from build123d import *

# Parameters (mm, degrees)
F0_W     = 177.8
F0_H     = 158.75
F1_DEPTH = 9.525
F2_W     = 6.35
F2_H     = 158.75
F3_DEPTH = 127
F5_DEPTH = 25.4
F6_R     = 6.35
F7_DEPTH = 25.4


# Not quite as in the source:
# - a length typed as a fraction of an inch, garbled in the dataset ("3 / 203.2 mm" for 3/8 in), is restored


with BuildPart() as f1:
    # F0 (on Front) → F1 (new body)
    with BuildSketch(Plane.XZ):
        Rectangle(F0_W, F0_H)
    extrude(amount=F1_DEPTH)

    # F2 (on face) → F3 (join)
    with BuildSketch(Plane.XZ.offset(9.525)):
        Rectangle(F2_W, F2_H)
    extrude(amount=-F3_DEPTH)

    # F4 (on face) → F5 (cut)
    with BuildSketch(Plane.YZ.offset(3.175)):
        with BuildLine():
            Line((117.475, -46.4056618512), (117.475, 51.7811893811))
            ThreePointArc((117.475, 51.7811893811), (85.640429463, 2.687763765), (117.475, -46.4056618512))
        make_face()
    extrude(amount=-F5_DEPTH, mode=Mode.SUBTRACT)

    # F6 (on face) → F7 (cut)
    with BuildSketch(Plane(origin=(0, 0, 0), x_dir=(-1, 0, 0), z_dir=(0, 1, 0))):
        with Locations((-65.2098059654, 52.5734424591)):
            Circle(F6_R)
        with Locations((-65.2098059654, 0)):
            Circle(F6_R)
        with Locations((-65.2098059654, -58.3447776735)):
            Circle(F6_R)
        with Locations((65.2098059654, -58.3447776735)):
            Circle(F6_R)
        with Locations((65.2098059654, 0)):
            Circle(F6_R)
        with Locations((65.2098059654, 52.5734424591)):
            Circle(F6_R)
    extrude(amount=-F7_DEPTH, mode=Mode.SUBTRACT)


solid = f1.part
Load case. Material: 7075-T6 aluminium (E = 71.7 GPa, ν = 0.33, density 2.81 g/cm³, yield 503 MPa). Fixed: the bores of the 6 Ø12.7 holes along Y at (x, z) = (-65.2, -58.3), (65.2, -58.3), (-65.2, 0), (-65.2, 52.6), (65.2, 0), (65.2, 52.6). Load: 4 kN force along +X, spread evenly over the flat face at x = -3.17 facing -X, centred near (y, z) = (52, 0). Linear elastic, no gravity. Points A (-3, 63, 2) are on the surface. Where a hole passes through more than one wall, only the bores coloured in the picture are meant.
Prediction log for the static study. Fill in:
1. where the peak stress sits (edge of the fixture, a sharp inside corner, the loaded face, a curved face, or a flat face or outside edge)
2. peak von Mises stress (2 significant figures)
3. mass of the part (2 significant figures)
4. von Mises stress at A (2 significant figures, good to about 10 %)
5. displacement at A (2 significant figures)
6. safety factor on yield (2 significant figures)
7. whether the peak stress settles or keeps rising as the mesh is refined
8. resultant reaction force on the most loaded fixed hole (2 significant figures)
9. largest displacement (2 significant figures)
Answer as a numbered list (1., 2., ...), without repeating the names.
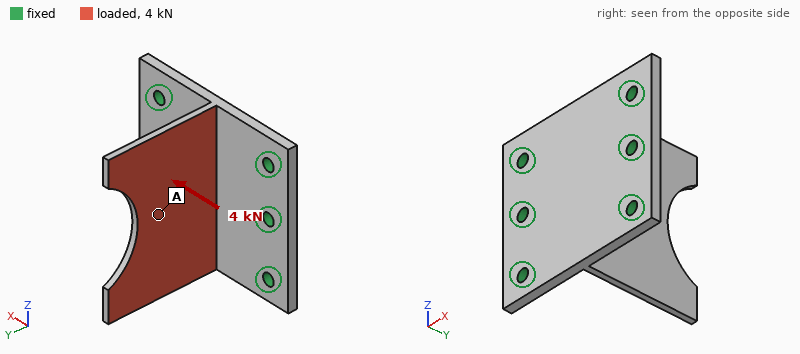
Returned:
1. a flat face or outside edge
2. 160 MPa
3. 1.0 kg
4. 26 MPa
5. 1.3 mm
6. 3.1
7. settles
8. 1.2 kN
9. 3.0 mm
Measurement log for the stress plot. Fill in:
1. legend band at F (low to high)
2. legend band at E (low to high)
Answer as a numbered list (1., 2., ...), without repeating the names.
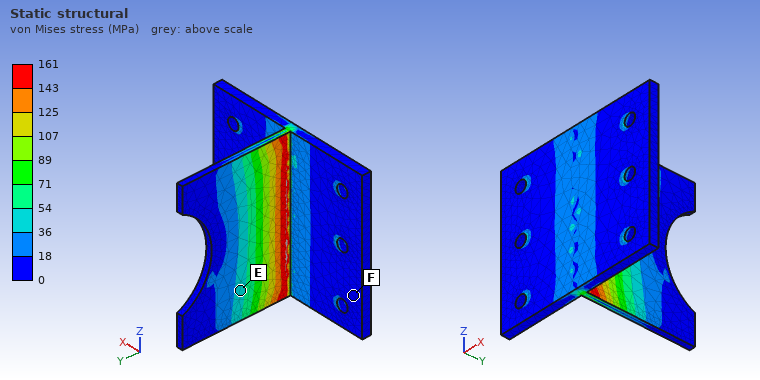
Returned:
1. 0 to 18 MPa
2. 36 to 54 MPa
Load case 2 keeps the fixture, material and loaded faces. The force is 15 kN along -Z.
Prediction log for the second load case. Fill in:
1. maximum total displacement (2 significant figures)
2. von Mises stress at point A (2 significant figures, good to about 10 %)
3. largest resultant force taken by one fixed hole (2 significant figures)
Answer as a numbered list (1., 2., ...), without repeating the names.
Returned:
1. 0.78 mm
2. 30 MPa
3. 4.7 kN
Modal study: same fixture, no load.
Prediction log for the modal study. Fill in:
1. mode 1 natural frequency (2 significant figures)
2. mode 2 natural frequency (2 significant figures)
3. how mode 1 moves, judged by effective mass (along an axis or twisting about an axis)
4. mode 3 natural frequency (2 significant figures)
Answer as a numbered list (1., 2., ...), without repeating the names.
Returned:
1. 450 Hz
2. 680 Hz
3. along X
4. 1400 Hz
